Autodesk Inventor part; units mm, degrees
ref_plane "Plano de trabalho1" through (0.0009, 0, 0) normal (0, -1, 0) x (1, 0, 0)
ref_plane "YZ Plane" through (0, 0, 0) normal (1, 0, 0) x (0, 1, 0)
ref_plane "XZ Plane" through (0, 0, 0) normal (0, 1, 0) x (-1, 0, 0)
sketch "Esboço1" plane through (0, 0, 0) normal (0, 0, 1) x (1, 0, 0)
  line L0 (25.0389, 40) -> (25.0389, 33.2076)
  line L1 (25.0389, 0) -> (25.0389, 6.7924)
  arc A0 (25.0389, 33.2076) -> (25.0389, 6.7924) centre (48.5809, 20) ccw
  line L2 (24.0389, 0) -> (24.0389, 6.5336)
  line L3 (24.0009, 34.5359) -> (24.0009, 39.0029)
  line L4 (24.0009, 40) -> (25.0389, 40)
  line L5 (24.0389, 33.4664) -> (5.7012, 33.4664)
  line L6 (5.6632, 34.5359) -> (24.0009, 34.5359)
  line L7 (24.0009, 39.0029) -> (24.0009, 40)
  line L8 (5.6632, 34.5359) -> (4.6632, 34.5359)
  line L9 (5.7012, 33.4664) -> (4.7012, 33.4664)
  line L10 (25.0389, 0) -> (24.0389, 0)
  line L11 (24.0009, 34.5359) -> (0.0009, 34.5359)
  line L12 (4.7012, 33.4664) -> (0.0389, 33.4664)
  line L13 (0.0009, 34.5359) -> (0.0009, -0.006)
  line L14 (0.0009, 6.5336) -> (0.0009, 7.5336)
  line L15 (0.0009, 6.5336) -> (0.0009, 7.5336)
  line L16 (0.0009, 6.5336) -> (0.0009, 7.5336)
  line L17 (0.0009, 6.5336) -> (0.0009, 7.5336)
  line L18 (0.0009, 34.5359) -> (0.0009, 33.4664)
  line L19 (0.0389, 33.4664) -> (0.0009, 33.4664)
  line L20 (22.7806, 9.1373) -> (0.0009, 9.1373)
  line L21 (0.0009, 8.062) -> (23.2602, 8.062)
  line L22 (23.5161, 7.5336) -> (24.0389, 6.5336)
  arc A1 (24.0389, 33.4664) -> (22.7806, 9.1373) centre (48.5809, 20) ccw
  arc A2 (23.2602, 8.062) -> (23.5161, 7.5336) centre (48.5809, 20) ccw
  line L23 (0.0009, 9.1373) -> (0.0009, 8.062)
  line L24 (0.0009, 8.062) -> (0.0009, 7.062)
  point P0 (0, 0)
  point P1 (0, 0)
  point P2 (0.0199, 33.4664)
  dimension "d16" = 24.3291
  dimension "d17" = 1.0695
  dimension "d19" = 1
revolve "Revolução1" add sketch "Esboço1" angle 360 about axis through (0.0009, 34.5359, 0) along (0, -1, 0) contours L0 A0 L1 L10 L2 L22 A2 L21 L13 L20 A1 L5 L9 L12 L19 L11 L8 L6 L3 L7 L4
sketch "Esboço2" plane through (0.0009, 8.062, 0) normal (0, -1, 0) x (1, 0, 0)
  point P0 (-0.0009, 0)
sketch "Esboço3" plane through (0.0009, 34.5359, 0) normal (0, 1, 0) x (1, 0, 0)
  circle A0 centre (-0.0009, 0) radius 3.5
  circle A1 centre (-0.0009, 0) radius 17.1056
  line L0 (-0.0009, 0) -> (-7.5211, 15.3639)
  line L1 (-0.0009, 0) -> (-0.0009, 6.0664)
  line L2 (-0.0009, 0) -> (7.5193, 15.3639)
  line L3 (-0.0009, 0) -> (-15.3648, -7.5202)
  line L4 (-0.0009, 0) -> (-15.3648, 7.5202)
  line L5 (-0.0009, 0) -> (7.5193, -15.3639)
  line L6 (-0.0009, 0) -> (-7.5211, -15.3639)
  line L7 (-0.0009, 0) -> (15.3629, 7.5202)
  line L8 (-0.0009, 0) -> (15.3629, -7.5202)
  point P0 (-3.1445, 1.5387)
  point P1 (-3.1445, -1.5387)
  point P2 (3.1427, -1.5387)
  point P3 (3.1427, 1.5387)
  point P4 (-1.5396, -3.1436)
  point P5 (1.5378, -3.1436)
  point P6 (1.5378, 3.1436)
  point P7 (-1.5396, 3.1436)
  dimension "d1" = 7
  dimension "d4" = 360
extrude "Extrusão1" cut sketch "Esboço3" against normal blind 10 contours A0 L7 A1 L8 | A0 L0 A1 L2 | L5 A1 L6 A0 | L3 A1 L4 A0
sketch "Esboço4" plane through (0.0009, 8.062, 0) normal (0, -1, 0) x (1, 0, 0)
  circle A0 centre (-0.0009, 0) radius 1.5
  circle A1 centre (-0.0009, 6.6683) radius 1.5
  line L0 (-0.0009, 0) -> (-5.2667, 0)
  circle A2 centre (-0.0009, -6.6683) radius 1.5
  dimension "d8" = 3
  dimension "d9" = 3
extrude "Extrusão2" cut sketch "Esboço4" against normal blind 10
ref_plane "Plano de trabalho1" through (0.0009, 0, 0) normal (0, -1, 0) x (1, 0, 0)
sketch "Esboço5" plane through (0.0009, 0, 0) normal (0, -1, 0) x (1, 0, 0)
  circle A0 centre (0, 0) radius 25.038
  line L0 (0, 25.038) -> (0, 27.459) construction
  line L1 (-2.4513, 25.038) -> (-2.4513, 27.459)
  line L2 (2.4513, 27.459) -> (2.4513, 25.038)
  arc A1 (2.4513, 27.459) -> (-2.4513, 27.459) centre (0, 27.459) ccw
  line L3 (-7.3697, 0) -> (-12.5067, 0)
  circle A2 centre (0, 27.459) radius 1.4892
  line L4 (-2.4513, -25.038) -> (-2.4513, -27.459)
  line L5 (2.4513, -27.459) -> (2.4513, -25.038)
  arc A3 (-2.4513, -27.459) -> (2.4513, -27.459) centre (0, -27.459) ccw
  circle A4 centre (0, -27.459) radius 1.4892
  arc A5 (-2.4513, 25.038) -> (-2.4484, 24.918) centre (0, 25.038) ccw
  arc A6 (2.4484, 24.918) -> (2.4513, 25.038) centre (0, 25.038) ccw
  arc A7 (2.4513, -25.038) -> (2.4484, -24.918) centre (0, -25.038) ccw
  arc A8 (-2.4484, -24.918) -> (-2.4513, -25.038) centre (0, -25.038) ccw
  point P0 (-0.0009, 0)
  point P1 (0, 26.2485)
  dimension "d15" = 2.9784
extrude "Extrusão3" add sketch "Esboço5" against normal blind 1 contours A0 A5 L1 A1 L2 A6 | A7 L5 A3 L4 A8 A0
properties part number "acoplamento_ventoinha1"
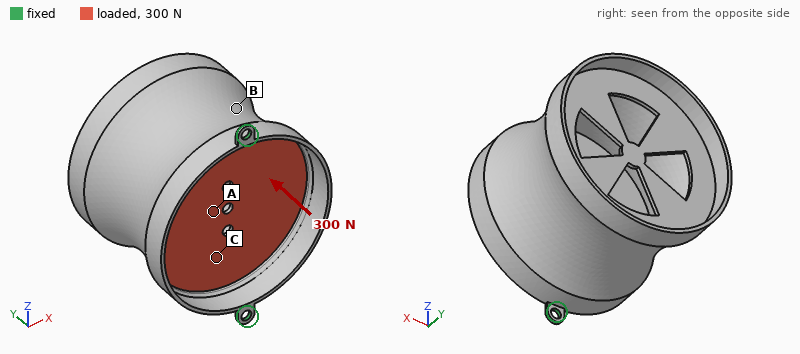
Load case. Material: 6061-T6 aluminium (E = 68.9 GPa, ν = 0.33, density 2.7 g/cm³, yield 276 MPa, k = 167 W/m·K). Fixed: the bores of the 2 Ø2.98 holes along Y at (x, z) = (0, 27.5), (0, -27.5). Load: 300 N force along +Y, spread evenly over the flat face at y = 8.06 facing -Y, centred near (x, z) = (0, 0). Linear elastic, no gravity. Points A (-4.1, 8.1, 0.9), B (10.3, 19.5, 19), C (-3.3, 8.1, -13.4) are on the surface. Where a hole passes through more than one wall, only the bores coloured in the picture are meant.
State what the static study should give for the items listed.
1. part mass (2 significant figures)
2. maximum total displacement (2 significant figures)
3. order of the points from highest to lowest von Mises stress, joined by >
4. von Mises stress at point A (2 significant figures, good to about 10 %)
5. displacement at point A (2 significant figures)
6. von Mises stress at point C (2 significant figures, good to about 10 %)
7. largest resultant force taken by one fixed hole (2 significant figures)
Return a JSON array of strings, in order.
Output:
["25 g", "0.14 mm", "A > C > B", "40 MPa", "0.13 mm", "22 MPa", "160 N"]
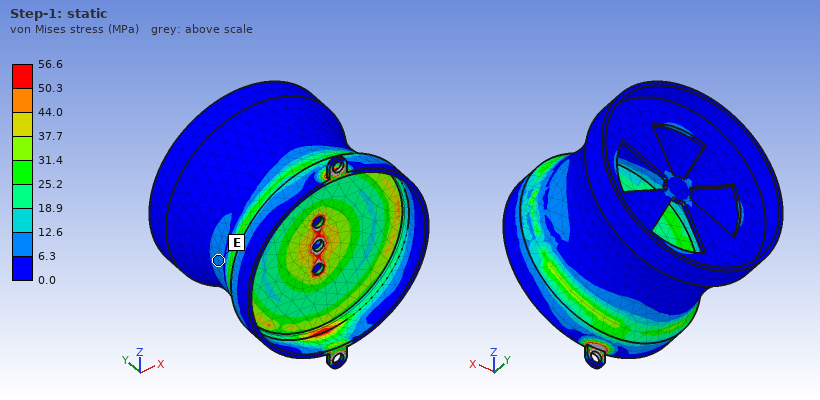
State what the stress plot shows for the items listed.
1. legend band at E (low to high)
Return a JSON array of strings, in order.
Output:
["6.3 to 12.6 MPa"]
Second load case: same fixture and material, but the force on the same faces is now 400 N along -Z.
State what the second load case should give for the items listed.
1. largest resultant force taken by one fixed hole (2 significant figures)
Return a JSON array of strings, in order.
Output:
["210 N"]
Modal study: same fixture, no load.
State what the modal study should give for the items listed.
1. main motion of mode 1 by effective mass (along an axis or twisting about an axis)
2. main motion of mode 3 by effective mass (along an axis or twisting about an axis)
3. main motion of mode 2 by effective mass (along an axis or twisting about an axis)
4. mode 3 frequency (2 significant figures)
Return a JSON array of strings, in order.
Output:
["along X", "along Y", "along Z", "3800 Hz"]
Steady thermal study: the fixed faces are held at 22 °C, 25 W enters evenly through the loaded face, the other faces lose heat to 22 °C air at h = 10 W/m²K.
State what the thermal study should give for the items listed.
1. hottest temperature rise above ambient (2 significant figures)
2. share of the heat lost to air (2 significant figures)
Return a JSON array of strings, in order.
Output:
["63 K", "33 %"]
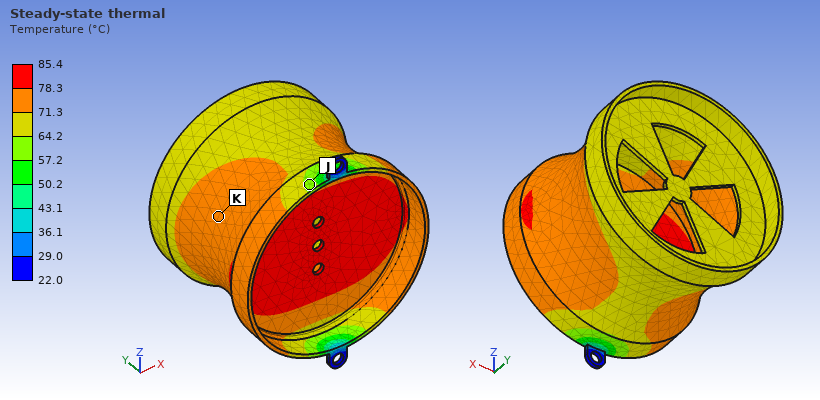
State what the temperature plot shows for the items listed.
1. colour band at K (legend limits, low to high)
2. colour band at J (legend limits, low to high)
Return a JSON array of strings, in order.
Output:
["71.3 to 78.3 °C", "57.2 to 64.2 °C"]
